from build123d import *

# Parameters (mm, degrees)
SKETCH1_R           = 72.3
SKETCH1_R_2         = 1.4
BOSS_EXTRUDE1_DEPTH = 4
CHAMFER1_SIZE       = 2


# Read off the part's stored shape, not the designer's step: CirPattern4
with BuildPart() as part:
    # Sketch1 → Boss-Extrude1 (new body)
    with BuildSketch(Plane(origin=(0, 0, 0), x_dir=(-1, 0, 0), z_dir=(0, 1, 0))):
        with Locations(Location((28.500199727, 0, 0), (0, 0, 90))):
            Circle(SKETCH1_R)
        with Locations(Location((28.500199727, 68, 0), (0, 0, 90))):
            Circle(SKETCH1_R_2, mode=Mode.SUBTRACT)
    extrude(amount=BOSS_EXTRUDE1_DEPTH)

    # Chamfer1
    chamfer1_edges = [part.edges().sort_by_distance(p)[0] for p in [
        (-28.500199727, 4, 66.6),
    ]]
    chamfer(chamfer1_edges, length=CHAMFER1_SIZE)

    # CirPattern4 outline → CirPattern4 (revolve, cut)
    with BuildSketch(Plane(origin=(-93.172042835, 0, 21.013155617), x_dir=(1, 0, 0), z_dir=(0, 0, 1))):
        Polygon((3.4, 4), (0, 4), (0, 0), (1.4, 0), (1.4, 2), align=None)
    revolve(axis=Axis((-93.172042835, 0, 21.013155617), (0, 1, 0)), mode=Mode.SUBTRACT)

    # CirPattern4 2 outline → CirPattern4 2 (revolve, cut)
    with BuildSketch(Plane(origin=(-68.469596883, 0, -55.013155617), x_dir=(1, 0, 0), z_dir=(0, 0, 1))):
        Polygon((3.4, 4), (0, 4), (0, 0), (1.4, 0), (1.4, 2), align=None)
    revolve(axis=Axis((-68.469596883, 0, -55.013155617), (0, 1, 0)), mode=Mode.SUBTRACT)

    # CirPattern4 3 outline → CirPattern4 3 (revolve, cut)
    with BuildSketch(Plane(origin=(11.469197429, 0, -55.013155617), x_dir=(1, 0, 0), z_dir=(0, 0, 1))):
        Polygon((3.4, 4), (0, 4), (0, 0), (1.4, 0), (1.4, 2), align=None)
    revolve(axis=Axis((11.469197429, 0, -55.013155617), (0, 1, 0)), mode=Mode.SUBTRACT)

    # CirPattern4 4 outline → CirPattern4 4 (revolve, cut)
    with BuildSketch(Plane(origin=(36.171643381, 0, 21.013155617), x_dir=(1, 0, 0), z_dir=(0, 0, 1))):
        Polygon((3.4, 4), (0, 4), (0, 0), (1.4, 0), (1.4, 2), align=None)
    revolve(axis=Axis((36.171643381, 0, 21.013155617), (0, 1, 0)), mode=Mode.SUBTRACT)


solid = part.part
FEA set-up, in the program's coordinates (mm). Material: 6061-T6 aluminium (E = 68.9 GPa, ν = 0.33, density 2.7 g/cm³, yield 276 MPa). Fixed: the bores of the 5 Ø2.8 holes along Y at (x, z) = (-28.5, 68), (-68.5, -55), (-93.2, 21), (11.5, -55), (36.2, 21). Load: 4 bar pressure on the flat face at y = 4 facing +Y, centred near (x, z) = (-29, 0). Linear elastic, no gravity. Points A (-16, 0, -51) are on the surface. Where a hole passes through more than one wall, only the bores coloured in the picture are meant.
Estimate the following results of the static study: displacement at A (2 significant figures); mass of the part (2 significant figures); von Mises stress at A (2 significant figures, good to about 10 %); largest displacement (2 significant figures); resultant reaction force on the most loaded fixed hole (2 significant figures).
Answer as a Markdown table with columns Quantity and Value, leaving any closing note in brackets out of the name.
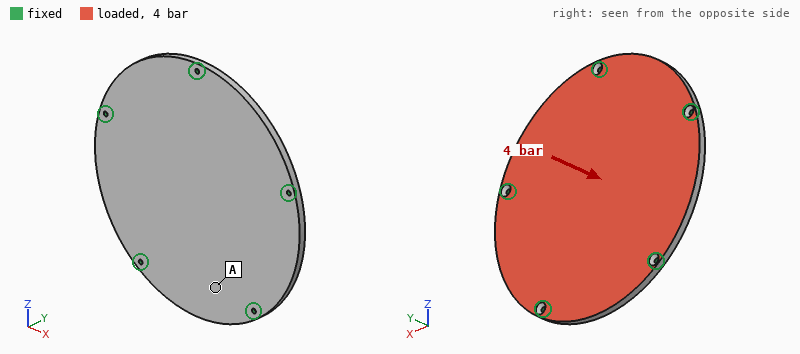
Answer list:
| Quantity | Value |
|---|---|
| displacement at A | 0.32 mm |
| mass of the part | 180 g |
| von Mises stress at A | 58 MPa |
| largest displacement | 0.80 mm |
| resultant reaction force on the most loaded fixed hole | 2.2 kN |
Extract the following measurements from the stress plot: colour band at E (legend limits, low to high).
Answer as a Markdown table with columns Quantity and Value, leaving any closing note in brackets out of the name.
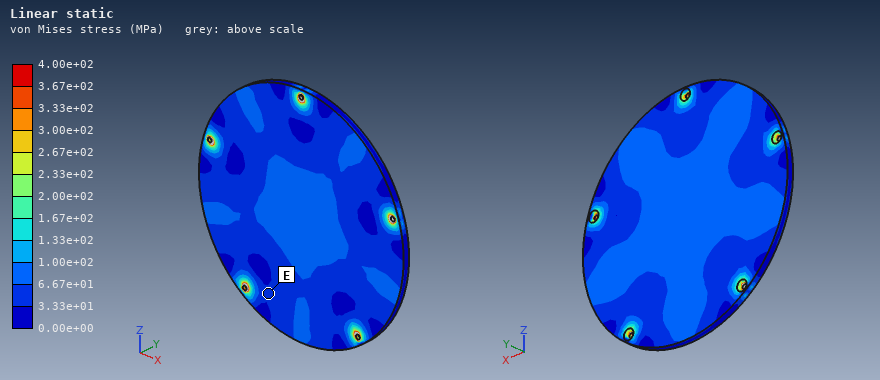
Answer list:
| Quantity | Value |
|---|---|
| colour band at E | 3.33e+01 to 6.67e+01 MPa |
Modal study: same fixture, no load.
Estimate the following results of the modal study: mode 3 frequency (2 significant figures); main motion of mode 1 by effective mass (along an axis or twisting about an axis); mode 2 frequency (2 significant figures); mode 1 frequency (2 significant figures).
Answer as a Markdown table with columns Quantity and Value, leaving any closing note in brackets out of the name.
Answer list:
| Quantity | Value |
|---|---|
| mode 3 frequency | 2400 Hz |
| main motion of mode 1 by effective mass | along Y |
| mode 2 frequency | 2400 Hz |
| mode 1 frequency | 1300 Hz |
